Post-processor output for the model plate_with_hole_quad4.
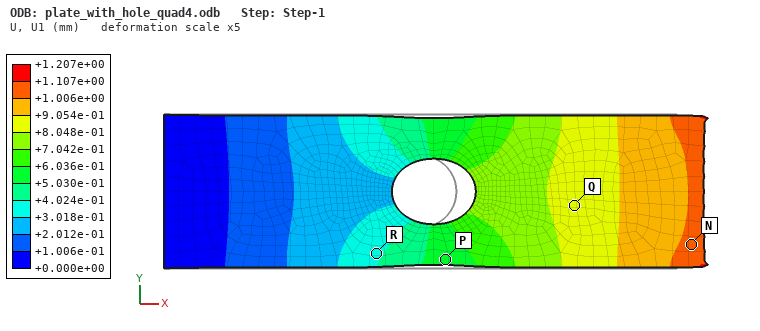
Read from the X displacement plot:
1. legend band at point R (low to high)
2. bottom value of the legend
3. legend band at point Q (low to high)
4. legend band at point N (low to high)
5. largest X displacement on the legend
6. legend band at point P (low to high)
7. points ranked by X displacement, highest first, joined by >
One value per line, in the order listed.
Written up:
+3.018e-01 to +4.024e-01 mm
+0.000e+00 mm
+8.048e-01 to +9.054e-01 mm
+1.006e+00 to +1.107e+00 mm
+1.207e+00 mm
+5.030e-01 to +6.036e-01 mm
N > Q > P > R
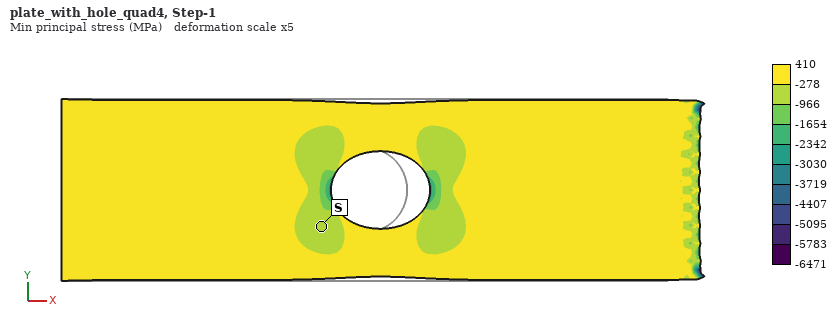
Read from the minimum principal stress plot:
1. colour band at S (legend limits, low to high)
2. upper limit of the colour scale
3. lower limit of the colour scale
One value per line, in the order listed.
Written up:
-966 to -278 MPa
410 MPa
-6471 MPa
